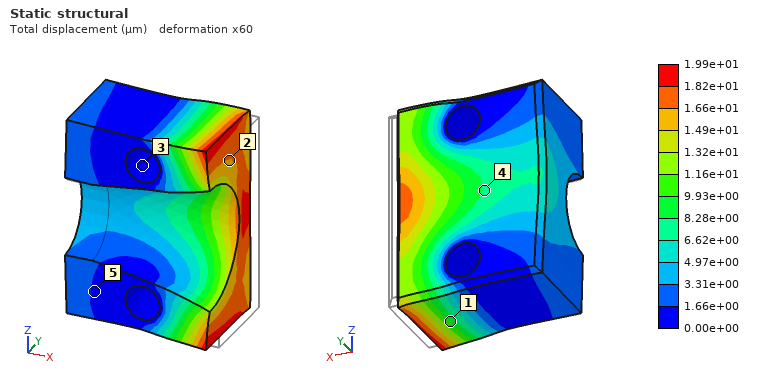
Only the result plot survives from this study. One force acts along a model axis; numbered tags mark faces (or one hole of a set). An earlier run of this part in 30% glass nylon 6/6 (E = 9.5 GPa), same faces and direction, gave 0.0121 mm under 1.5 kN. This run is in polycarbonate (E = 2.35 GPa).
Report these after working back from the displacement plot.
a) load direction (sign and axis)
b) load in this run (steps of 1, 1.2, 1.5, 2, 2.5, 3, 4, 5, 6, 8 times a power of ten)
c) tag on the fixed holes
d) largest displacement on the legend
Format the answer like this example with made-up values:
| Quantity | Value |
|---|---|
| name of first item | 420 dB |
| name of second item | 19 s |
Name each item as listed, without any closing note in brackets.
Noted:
| Quantity | Value |
|---|---|
| load direction | -X |
| load in this run | 600 N |
| tag on the fixed holes | 3 |
| largest displacement on the legend | 1.99e+01 µm |
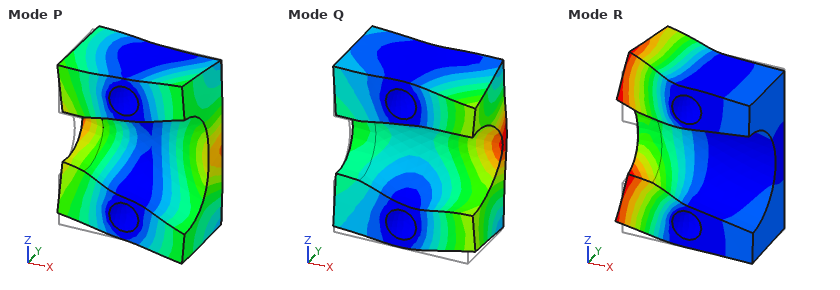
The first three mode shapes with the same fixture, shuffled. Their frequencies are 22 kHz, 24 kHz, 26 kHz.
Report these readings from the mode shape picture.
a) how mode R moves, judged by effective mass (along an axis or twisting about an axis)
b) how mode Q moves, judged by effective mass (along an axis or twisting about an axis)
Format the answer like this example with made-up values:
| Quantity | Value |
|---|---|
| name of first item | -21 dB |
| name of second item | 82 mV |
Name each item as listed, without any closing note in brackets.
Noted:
| Quantity | Value |
|---|---|
| how mode R moves, judged by effective mass | along Z |
| how mode Q moves, judged by effective mass | along Y |
